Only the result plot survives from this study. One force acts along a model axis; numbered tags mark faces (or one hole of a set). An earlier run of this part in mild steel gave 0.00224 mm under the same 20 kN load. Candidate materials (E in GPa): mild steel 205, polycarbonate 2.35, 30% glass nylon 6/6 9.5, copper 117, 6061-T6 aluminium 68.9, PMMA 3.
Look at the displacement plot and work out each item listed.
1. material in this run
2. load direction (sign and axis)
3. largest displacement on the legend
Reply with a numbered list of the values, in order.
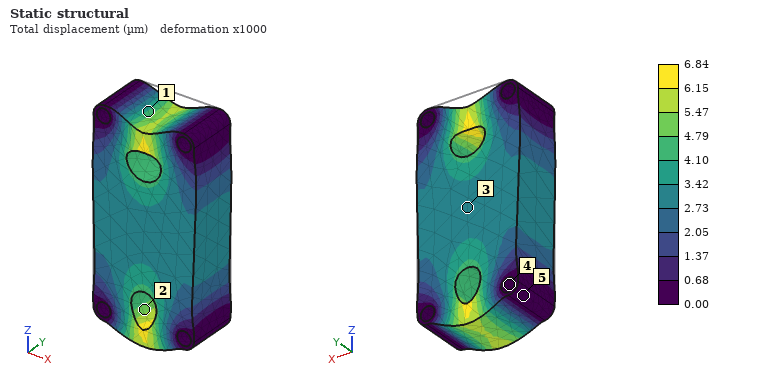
1. 6061-T6 aluminium
2. -Z
3. 6.84 µm
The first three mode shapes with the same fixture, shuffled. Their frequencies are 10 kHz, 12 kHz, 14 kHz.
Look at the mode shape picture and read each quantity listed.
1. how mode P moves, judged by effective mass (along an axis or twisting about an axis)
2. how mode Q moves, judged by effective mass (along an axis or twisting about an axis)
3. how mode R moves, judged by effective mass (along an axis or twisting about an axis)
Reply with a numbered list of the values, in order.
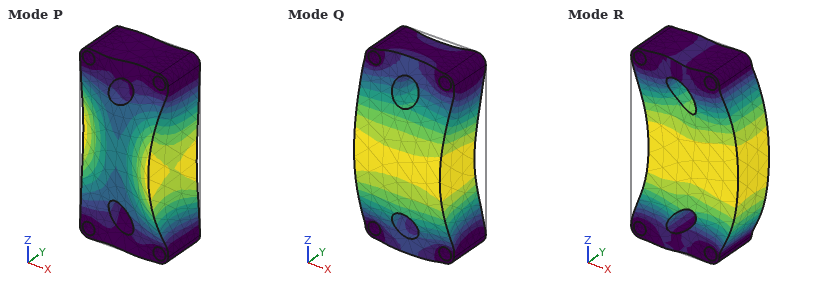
1. twisting about Z
2. along Y
3. along X
